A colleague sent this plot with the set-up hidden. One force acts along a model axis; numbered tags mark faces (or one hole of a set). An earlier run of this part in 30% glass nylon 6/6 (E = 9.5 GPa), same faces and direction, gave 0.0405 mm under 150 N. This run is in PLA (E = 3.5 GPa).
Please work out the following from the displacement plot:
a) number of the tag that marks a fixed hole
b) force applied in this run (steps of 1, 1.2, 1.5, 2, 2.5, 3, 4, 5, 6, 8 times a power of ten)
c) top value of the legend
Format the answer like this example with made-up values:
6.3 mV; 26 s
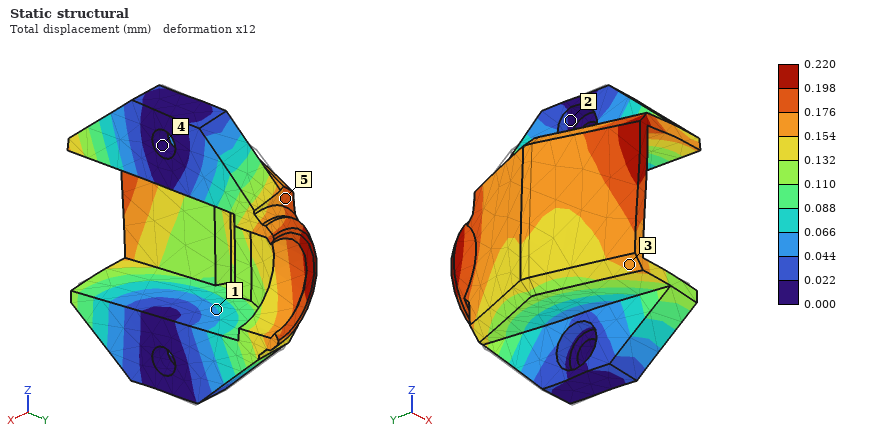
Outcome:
4; 300 N; 0.220 mm
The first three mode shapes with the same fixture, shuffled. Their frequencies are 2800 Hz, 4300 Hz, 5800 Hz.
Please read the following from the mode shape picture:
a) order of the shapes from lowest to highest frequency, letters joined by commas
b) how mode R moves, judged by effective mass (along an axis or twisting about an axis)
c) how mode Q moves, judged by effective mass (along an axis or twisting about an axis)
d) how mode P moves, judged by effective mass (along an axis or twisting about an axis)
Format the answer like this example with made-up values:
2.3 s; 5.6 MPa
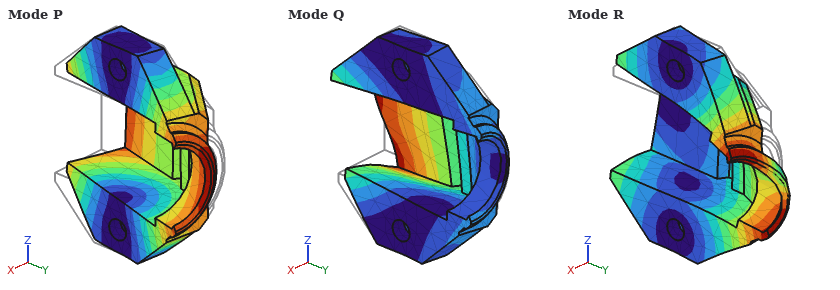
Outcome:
P, Q, R; along Z; along Z; along Y
